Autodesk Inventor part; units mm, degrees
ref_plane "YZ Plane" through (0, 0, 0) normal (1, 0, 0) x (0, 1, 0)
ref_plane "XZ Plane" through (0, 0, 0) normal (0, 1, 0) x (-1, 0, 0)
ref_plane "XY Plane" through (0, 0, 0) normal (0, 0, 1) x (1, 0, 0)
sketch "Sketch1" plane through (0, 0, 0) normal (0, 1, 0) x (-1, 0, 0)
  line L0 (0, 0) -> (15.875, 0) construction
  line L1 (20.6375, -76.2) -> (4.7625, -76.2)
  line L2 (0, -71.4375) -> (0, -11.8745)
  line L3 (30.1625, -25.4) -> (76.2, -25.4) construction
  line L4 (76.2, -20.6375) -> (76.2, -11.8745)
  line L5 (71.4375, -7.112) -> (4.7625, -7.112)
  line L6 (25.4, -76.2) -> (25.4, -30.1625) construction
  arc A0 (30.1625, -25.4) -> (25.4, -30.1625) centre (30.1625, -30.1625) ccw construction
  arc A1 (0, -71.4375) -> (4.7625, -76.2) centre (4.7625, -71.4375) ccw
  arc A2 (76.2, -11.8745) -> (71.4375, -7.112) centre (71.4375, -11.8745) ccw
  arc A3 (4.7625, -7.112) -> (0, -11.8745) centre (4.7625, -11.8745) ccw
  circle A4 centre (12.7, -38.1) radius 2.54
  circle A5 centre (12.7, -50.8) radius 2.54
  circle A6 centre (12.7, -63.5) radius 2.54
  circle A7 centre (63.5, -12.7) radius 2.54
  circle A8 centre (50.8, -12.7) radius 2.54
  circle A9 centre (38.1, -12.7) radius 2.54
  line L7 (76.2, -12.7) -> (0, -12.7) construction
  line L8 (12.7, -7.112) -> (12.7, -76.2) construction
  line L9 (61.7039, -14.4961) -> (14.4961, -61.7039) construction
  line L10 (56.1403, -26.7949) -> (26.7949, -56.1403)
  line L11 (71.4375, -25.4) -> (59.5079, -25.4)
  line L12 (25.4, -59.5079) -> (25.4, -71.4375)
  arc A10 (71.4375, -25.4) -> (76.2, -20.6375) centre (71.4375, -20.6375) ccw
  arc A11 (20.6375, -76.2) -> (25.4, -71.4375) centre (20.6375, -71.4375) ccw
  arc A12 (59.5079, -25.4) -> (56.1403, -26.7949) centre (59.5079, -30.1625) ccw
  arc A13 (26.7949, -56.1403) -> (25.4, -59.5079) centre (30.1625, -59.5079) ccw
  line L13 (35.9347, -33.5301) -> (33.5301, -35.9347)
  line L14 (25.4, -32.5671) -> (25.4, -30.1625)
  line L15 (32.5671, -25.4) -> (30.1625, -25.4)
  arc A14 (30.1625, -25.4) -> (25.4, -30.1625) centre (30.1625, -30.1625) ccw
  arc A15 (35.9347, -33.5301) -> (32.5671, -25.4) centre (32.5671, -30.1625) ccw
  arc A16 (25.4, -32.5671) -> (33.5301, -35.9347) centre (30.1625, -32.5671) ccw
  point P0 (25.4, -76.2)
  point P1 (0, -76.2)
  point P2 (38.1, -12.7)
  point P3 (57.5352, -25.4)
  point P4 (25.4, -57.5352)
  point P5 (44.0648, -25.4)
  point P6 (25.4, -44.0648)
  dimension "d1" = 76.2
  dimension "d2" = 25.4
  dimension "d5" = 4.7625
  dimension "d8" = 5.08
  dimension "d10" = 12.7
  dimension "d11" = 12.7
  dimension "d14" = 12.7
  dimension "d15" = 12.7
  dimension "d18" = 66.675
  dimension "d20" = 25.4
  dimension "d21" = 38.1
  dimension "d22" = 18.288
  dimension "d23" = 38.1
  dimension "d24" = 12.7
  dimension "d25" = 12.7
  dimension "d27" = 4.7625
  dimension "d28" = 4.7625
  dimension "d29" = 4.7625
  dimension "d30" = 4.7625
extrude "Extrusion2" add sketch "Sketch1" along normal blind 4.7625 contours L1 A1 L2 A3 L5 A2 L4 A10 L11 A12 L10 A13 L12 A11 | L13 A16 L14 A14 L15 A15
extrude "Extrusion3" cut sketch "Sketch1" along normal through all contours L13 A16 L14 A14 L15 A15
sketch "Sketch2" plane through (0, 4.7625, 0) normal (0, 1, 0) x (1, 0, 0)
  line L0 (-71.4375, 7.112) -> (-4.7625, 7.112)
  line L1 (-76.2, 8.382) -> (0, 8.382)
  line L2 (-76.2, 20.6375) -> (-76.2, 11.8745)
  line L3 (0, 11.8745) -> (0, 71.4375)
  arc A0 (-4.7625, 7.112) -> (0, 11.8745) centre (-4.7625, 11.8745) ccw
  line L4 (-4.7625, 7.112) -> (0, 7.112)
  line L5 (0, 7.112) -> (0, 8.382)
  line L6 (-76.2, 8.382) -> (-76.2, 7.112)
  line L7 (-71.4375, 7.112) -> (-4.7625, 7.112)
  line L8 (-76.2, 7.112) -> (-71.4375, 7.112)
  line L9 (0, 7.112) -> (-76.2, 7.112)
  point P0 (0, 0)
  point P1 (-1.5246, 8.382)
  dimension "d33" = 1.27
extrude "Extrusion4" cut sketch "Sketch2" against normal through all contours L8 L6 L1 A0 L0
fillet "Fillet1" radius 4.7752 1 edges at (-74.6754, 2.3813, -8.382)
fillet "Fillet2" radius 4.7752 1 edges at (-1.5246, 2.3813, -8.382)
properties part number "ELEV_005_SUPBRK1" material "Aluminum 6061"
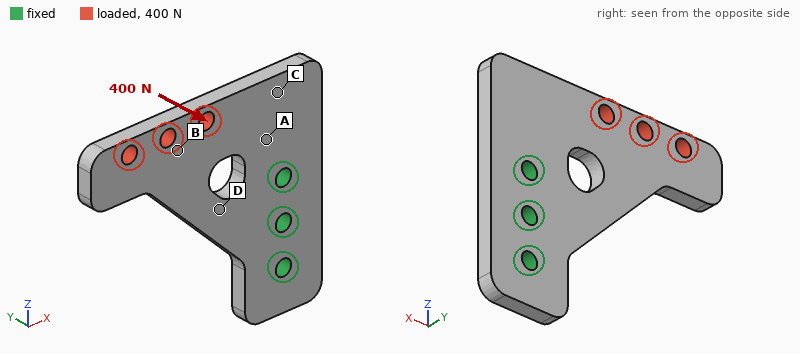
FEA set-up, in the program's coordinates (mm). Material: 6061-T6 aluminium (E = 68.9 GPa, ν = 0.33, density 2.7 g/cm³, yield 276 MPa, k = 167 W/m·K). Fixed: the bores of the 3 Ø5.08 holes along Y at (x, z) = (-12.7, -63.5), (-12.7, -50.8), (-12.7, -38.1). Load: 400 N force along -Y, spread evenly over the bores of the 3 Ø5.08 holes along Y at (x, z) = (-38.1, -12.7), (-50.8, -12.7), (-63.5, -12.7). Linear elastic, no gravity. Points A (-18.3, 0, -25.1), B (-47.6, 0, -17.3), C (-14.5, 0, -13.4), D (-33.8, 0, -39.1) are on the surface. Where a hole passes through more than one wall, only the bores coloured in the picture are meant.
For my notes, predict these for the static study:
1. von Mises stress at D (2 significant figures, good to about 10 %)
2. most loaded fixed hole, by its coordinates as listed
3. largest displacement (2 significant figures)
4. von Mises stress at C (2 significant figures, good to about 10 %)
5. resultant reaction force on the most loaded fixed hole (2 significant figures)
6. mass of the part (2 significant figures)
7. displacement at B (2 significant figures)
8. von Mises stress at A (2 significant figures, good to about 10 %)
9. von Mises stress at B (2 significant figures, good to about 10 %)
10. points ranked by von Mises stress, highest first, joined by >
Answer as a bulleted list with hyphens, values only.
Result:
- 120 MPa
- (-12.7, -38.1)
- 1.2 mm
- 64 MPa
- 670 N
- 37 g
- 0.53 mm
- 90 MPa
- 39 MPa
- D > A > C > B
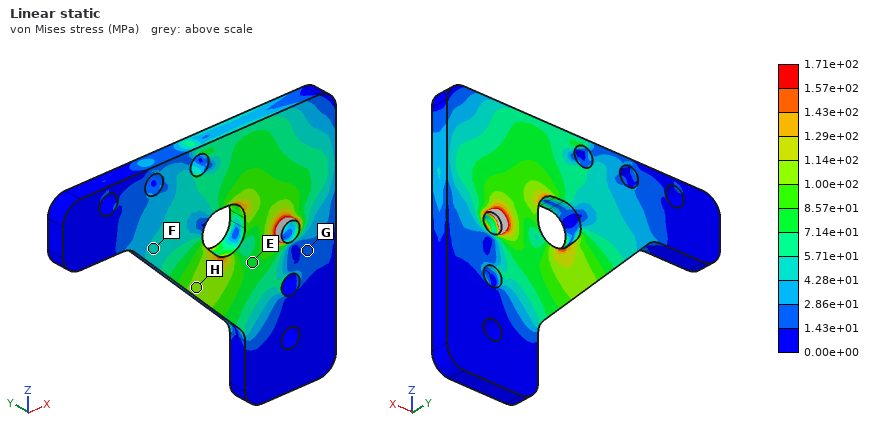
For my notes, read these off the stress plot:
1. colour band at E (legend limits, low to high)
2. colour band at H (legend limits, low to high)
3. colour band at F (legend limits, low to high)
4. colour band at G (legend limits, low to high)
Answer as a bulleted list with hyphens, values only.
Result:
- 7.14e+01 to 8.57e+01 MPa
- 1.00e+02 to 1.14e+02 MPa
- 4.28e+01 to 5.71e+01 MPa
- 1.43e+01 to 2.86e+01 MPa
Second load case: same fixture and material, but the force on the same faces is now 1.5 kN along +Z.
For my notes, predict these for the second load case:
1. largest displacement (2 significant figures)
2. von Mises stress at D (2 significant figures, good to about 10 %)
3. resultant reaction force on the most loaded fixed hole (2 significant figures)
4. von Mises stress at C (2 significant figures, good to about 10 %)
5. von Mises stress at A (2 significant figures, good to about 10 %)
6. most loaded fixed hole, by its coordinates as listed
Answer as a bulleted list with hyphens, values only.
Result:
- 0.12 mm
- 37 MPa
- 2.4 kN
- 11 MPa
- 19 MPa
- (-12.7, -38.1)
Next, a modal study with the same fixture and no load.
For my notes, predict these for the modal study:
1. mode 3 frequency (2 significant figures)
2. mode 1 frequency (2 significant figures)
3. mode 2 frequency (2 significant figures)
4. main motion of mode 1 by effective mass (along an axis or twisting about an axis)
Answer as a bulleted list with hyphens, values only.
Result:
- 5500 Hz
- 1100 Hz
- 3800 Hz
- along Y
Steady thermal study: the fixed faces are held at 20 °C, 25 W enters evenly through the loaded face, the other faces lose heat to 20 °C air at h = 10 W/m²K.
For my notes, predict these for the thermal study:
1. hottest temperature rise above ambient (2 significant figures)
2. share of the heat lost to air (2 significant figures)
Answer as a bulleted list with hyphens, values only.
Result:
- 57 K
- 5.3 %
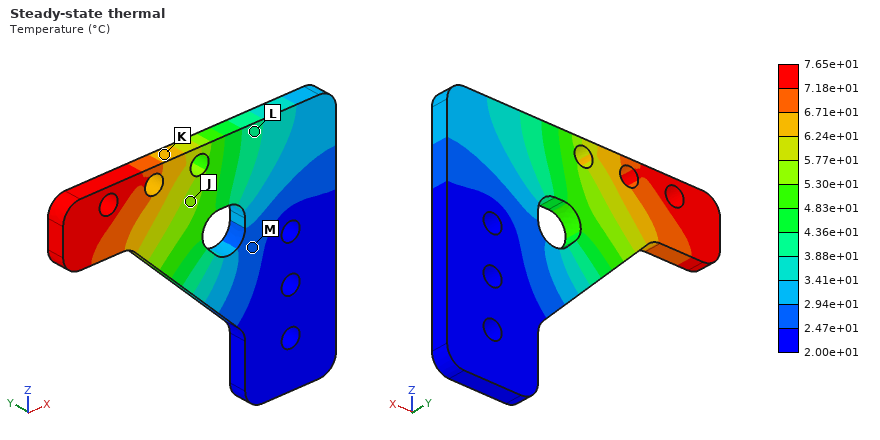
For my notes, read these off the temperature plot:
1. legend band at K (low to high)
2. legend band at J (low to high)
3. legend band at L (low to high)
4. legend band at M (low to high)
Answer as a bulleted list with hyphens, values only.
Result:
- 6.24e+01 to 6.71e+01 °C
- 5.30e+01 to 5.77e+01 °C
- 3.88e+01 to 4.36e+01 °C
- 2.47e+01 to 2.94e+01 °C
